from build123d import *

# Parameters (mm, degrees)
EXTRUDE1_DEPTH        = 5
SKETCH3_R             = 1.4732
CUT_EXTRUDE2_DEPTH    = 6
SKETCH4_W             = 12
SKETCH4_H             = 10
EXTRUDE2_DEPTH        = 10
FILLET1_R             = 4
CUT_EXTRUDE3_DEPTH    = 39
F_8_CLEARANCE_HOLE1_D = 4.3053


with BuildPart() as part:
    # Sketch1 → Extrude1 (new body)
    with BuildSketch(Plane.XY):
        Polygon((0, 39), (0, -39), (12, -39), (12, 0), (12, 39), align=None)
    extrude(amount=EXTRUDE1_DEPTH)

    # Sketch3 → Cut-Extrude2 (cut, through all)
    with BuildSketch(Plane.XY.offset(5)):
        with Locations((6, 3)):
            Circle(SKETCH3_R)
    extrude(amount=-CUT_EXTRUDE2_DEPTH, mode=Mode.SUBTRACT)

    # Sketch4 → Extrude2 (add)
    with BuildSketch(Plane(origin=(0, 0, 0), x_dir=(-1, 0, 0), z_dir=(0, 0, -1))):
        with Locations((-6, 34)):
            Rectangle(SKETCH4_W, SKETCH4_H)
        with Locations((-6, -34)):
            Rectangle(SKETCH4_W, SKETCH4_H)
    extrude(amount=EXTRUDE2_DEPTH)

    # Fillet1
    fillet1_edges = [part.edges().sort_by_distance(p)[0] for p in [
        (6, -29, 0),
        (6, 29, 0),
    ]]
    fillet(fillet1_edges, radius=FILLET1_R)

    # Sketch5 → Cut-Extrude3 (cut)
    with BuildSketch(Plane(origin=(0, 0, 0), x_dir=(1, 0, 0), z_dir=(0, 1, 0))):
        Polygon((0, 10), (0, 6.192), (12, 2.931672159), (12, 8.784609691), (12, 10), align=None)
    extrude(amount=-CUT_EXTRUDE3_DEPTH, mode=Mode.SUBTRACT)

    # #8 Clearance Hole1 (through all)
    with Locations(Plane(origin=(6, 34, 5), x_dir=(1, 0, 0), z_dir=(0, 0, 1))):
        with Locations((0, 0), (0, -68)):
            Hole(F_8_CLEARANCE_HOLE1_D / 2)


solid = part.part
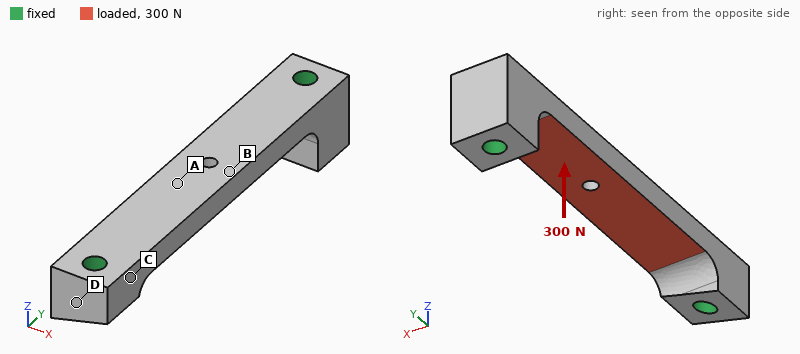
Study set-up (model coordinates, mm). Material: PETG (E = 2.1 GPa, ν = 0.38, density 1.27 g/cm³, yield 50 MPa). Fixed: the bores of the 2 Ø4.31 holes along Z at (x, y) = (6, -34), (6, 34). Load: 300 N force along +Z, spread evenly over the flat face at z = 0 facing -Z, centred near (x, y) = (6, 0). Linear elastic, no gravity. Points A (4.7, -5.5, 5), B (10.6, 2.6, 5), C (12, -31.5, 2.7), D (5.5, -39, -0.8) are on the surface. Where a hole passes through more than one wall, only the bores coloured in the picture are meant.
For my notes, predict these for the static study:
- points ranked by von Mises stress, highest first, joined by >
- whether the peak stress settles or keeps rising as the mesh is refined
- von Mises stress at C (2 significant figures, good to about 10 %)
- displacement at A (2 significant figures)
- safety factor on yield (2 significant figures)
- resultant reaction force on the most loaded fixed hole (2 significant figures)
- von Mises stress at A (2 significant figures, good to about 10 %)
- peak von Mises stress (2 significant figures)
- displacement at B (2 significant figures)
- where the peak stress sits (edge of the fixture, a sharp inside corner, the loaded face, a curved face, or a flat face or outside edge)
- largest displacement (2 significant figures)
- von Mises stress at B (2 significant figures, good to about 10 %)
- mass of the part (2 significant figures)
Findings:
B > A > C > D
settles
5.7 MPa
0.73 mm
1.3
160 N
16 MPa
39 MPa
0.78 mm
a curved face
0.81 mm
20 MPa
7.8 g
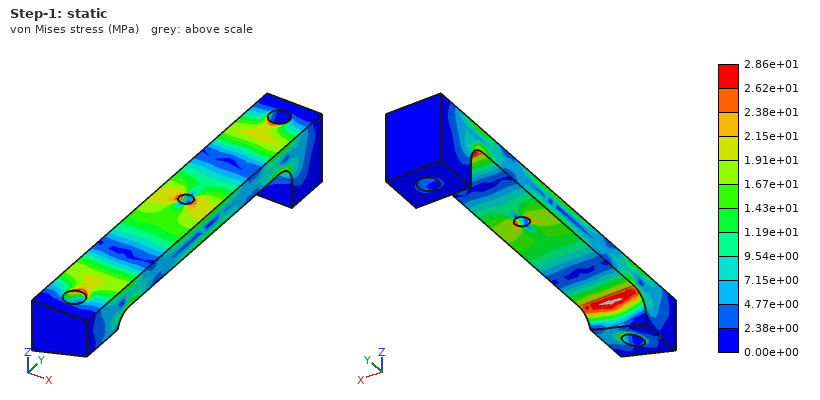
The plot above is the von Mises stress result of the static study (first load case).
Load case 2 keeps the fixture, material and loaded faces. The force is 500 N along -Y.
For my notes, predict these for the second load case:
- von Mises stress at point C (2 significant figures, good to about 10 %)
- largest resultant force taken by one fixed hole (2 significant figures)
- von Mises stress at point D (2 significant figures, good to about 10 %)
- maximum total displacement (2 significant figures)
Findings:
2.0 MPa
250 N
1.00 MPa
49 µm
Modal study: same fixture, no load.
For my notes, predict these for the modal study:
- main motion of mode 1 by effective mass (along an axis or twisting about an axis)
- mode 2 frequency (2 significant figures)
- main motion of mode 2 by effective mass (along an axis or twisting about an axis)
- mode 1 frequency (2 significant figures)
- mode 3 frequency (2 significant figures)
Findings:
along Z
2900 Hz
along X
1800 Hz
4600 Hz
